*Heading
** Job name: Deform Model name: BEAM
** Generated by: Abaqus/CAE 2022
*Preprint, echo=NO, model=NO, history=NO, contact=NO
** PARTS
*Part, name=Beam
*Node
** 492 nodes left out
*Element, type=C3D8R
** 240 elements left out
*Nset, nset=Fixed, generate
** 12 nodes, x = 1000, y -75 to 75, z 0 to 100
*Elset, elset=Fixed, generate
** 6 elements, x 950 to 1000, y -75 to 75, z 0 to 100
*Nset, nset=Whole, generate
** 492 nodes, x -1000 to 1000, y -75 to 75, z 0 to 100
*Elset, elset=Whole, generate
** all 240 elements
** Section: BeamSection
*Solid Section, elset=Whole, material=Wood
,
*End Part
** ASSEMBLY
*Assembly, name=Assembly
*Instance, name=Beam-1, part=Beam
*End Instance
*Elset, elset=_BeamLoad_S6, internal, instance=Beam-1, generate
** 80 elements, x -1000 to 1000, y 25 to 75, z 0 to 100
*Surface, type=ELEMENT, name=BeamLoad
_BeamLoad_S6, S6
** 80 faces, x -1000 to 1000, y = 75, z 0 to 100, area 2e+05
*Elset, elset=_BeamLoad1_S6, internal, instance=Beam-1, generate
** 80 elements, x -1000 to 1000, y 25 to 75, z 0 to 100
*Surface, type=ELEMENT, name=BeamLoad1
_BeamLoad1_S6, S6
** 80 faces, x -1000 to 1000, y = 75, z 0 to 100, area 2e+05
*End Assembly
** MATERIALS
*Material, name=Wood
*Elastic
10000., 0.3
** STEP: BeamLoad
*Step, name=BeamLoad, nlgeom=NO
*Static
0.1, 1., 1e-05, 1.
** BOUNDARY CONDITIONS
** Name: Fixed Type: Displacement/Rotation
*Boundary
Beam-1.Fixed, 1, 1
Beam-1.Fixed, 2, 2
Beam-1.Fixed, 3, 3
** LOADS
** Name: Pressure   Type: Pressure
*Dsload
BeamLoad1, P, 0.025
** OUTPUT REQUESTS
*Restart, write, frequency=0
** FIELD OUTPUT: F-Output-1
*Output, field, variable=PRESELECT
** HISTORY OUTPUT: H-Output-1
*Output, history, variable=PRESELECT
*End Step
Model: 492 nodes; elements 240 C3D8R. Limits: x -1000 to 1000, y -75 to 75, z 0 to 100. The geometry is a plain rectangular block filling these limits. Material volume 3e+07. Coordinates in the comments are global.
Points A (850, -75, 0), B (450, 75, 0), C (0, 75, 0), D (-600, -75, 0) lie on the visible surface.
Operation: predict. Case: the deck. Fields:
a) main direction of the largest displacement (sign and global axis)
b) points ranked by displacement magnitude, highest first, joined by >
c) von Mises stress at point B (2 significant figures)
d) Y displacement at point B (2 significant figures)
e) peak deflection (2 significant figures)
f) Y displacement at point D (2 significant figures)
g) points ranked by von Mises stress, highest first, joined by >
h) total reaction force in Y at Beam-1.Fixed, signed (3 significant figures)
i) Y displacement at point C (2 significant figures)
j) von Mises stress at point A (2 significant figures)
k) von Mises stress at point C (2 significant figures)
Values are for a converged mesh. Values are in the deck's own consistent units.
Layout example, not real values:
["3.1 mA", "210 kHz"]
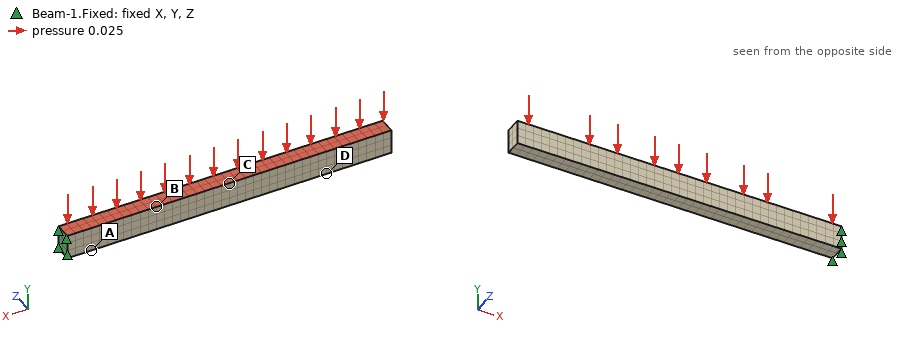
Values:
["-Y", "D > C > B > A", "7.0", "-2.3", "18", "-13", "A > B > C > D", "5000", "-6.3", "11", "3.3"]
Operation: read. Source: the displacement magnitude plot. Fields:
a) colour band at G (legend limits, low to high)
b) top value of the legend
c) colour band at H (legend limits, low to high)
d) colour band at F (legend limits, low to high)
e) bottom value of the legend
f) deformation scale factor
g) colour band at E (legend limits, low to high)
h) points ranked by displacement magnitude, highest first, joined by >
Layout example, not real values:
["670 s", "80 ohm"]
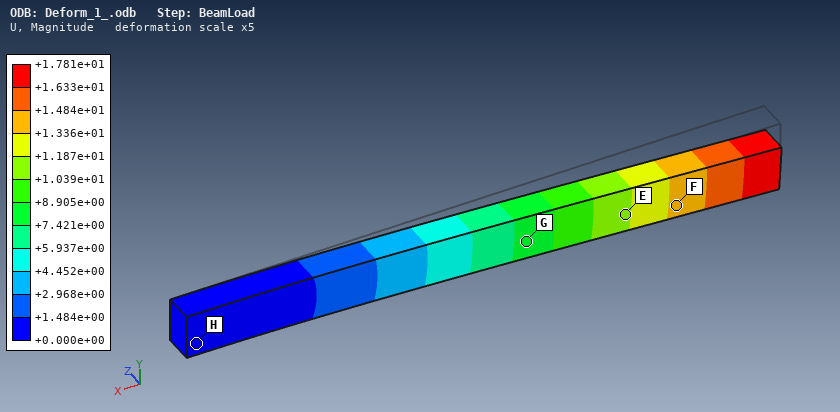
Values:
["+7.421e+00 to +8.905e+00", "+1.781e+01", "+0.000e+00 to +1.484e+00", "+1.336e+01 to +1.484e+01", "+0.000e+00", "5", "+1.039e+01 to +1.187e+01", "F > E > G > H"]
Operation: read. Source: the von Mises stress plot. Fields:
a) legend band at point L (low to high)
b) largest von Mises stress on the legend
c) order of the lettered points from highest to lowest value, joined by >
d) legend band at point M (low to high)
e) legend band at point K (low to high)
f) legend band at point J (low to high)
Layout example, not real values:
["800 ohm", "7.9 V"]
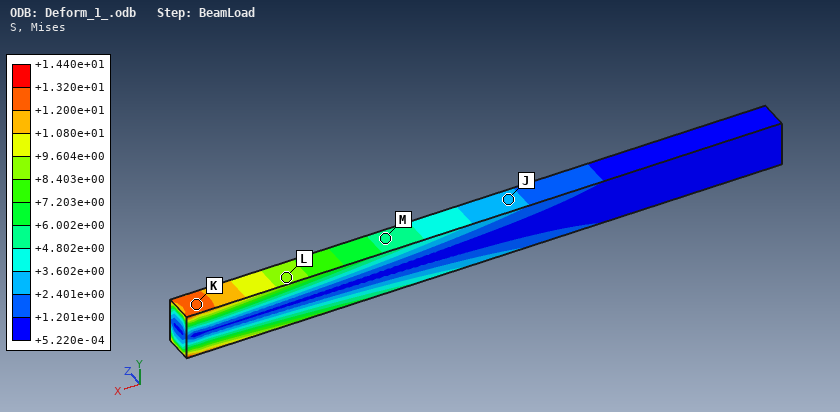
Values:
["+8.403e+00 to +9.604e+00", "+1.440e+01", "K > L > M > J", "+4.802e+00 to +6.002e+00", "+1.200e+01 to +1.320e+01", "+2.401e+00 to +3.602e+00"]
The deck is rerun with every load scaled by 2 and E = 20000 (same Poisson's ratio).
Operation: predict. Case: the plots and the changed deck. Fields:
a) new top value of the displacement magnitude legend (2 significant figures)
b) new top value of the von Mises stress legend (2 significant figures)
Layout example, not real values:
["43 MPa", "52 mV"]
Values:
["18", "29"]
